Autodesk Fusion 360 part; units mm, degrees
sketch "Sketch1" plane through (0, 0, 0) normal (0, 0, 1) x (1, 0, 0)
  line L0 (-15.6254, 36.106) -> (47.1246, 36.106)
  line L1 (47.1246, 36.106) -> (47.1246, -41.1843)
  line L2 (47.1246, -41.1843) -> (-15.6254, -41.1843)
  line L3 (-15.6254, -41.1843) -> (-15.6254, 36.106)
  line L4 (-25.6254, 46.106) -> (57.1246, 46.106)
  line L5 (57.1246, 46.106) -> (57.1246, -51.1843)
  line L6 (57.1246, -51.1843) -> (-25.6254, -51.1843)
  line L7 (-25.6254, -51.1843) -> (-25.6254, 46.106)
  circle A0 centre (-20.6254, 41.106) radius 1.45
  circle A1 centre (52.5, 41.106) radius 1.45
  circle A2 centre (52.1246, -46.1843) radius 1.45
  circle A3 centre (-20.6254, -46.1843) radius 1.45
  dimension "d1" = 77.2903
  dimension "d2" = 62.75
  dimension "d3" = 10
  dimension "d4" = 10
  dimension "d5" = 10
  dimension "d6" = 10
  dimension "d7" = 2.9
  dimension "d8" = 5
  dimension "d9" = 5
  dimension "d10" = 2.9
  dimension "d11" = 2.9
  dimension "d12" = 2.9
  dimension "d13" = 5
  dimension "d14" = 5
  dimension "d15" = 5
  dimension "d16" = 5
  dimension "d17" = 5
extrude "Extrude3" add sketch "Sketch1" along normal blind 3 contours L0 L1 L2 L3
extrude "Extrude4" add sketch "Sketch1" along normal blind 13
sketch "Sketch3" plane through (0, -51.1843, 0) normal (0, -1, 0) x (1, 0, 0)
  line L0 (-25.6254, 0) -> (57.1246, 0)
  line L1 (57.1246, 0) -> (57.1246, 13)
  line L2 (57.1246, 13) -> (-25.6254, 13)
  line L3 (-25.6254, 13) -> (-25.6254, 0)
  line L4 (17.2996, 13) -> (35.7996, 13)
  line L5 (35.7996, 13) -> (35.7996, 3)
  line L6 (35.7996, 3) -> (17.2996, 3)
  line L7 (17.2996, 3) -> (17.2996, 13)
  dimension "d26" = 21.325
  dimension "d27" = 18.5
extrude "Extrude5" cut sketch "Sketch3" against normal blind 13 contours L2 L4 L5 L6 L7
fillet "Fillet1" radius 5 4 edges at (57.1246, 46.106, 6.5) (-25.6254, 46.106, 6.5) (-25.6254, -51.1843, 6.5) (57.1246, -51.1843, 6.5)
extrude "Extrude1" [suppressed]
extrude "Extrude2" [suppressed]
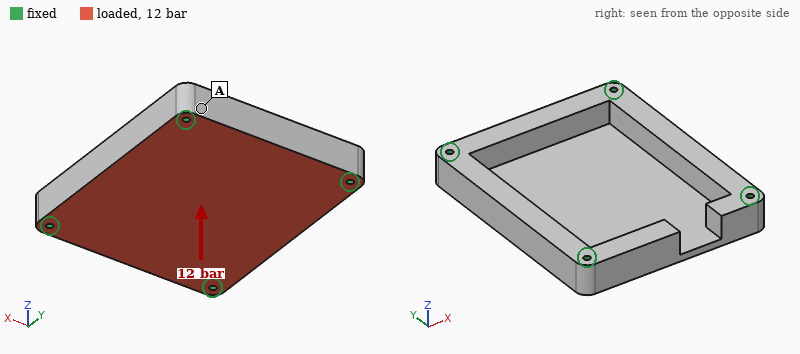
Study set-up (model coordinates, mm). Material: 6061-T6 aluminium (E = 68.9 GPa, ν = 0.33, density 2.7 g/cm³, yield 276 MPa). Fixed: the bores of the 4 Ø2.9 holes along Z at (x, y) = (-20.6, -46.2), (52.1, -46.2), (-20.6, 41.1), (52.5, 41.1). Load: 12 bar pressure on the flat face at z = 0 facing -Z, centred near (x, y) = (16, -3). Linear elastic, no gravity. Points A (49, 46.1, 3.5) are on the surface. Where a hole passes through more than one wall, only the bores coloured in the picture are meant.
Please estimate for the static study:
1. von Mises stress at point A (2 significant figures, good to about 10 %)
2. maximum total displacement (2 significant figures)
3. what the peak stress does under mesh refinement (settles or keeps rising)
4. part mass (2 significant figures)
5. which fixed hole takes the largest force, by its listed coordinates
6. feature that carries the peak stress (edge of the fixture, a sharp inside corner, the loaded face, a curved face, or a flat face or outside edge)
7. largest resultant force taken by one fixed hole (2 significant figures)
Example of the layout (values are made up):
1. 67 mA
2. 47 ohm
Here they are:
1. 22 MPa
2. 0.35 mm
3. keeps rising
4. 140 g
5. (-20.6, -46.2)
6. edge of the fixture
7. 3.4 kN
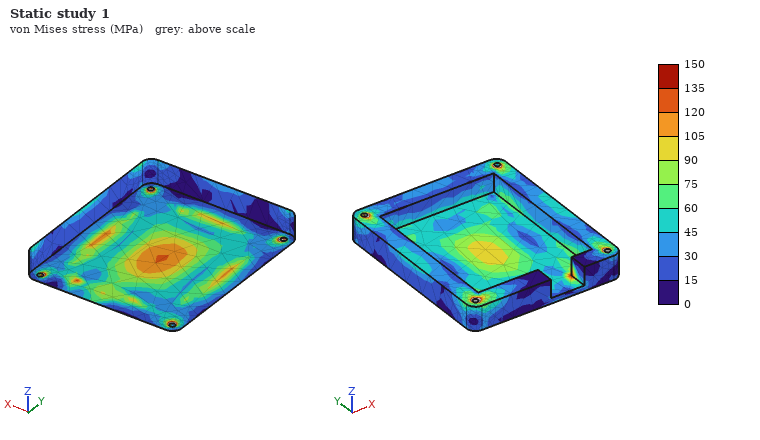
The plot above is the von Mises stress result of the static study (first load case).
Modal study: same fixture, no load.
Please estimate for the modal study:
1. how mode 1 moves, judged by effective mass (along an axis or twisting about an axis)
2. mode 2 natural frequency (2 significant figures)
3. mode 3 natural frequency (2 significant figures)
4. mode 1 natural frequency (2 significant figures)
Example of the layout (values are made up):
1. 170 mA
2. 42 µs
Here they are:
1. along Z
2. 6800 Hz
3. 6900 Hz
4. 4100 Hz
